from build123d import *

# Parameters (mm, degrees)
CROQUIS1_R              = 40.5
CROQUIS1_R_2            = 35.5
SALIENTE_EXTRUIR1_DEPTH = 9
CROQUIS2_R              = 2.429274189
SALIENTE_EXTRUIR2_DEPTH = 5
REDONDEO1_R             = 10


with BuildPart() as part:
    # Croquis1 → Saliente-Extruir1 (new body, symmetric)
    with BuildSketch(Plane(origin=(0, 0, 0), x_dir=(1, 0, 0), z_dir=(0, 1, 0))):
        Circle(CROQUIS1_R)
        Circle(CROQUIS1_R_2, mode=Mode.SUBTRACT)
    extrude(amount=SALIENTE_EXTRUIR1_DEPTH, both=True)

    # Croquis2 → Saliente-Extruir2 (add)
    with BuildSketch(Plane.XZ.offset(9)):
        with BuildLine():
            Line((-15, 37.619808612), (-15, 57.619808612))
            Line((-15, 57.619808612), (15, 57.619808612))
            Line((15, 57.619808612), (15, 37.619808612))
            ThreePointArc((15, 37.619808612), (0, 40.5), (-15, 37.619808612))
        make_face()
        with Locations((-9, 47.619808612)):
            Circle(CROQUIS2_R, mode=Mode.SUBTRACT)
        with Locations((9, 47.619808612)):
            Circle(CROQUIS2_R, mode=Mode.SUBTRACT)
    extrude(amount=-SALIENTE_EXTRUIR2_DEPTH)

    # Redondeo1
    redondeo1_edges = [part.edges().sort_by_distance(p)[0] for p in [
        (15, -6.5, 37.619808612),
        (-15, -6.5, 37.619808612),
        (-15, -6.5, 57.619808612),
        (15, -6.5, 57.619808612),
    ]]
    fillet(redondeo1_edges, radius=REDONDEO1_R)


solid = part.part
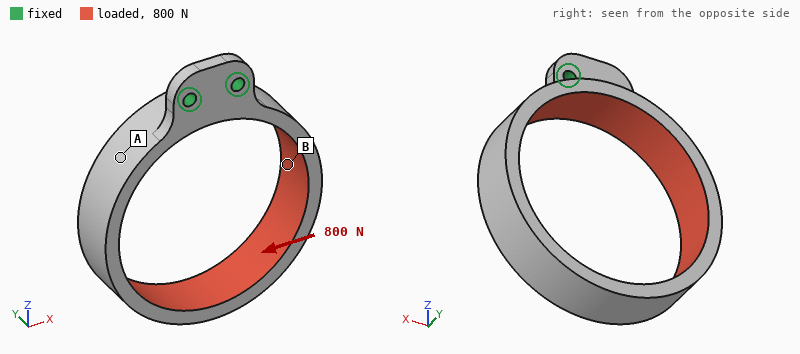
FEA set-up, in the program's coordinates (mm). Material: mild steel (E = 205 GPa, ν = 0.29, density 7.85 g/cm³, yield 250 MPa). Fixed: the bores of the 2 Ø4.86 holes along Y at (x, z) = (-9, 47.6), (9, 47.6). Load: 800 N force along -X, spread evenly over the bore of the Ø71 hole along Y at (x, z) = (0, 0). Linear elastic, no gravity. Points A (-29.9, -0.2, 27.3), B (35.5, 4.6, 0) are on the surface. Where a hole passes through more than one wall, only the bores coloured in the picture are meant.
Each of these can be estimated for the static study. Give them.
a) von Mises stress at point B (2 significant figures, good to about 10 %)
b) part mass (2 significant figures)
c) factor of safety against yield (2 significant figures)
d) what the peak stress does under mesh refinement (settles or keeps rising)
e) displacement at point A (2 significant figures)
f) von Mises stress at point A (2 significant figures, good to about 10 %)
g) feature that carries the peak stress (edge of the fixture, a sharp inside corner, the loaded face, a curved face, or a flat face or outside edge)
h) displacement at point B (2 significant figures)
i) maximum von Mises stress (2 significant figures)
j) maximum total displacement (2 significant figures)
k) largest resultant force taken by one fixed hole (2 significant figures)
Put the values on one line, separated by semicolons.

26 MPa; 190 g; 0.94; settles; 0.074 mm; 74 MPa; a curved face; 0.23 mm; 270 MPa; 0.39 mm; 1.8 kN
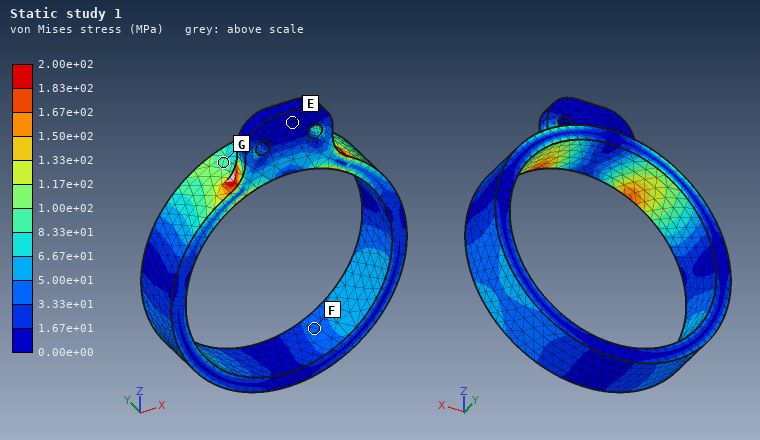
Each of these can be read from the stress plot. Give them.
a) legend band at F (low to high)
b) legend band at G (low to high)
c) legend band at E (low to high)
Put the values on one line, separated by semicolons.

3.33e+01 to 5.00e+01 MPa; 8.33e+01 to 1.00e+02 MPa; 0.00e+00 to 1.67e+01 MPa
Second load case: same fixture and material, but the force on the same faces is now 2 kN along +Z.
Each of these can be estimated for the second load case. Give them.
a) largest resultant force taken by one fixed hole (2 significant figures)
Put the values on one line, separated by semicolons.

1.2 kN
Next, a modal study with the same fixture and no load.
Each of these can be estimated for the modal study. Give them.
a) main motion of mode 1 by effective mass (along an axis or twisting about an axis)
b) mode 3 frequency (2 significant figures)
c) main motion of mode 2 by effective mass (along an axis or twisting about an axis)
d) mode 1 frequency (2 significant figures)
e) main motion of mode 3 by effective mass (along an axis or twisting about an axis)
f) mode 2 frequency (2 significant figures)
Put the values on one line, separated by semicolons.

along Y; 1500 Hz; along X; 480 Hz; twisting about Z; 600 Hz
